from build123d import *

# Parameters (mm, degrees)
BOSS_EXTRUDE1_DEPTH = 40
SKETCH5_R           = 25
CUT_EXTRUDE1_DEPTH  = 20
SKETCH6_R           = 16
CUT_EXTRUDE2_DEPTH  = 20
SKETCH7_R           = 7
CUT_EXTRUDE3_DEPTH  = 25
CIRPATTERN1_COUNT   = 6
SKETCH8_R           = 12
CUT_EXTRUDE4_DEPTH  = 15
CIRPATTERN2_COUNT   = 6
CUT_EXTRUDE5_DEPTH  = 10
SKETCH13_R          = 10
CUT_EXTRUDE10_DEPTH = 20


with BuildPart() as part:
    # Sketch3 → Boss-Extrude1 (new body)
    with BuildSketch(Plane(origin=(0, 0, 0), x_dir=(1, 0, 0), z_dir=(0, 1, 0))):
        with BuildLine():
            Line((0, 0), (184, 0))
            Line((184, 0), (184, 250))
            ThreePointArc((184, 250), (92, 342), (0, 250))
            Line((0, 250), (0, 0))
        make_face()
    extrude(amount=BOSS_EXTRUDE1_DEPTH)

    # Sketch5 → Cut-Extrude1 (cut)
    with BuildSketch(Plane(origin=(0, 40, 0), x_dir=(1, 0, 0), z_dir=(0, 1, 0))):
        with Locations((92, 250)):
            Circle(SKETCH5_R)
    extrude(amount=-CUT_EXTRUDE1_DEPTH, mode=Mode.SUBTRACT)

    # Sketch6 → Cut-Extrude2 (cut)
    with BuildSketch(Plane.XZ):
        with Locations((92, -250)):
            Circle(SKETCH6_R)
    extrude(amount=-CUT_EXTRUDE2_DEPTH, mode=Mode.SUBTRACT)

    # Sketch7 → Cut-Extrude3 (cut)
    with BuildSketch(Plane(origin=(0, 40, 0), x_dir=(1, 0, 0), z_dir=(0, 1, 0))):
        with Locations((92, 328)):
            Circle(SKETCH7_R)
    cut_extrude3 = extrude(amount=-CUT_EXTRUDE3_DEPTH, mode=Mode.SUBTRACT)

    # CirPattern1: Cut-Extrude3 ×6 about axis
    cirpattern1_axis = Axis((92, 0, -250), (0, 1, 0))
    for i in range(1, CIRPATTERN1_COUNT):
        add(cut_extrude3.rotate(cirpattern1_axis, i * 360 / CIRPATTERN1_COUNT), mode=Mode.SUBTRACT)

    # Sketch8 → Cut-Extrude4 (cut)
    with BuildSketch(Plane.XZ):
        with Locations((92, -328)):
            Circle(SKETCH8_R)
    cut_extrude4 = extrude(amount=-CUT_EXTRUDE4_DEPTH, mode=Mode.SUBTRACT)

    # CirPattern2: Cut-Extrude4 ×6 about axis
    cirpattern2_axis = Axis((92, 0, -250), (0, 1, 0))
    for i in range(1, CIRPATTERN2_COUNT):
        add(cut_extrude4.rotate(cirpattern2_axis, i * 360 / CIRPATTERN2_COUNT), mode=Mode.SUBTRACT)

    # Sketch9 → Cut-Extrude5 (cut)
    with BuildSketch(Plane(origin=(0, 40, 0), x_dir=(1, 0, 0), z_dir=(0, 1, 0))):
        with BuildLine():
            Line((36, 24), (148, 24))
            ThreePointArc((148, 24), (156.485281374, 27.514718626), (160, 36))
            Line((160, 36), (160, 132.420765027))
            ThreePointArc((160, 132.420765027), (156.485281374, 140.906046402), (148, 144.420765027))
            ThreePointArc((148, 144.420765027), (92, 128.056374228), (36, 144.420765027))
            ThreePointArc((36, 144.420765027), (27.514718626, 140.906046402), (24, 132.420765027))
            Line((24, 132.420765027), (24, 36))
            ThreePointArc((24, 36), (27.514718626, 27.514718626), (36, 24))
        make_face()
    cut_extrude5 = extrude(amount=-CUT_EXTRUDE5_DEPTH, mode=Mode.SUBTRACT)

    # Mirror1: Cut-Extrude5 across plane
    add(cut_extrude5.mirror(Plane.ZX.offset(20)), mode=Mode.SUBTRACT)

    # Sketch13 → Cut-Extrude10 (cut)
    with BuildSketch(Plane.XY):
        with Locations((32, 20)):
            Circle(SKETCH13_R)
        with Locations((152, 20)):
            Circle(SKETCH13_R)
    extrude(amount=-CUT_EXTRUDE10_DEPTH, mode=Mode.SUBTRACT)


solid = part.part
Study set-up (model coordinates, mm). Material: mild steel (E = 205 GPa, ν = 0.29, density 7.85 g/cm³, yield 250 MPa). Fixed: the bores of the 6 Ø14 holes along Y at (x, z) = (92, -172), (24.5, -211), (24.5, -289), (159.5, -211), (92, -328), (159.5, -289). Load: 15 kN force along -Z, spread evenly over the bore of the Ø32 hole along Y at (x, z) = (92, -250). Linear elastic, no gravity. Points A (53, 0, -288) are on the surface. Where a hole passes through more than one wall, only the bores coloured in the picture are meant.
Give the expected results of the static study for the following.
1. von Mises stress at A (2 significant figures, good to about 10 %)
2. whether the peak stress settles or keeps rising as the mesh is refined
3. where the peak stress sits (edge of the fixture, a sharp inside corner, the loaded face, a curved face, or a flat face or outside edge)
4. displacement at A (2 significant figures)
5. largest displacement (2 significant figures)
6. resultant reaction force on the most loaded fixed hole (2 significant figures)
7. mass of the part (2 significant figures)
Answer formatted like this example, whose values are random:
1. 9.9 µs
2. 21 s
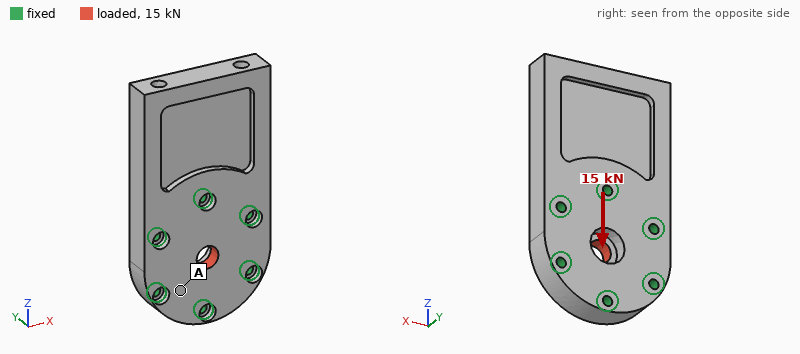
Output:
1. 1.7 MPa
2. keeps rising
3. a sharp inside corner
4. 0.54 µm
5. 1.7 µm
6. 3.7 kN
7. 15 kg
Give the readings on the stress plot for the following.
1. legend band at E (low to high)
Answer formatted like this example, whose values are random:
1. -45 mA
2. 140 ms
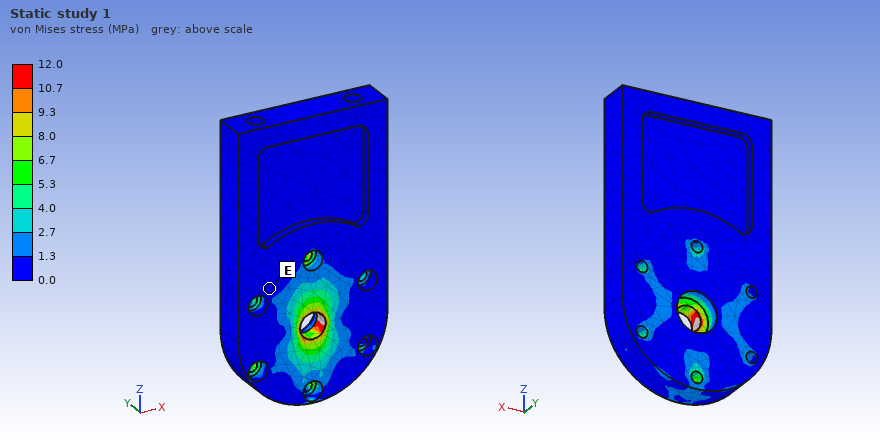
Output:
1. 0.0 to 1.3 MPa
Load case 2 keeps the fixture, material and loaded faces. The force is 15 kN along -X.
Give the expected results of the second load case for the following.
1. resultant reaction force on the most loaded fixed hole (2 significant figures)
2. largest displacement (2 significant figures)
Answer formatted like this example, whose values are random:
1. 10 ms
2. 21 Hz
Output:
1. 3.4 kN
2. 1.7 µm
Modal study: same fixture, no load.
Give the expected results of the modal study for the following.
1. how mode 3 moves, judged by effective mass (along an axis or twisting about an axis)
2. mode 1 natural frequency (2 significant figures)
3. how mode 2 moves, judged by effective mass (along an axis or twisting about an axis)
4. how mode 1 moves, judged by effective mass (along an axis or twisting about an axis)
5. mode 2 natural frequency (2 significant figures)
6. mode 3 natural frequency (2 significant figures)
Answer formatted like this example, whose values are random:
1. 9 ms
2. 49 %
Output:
1. along X
2. 750 Hz
3. twisting about Z
4. along Y
5. 1300 Hz
6. 2500 Hz
